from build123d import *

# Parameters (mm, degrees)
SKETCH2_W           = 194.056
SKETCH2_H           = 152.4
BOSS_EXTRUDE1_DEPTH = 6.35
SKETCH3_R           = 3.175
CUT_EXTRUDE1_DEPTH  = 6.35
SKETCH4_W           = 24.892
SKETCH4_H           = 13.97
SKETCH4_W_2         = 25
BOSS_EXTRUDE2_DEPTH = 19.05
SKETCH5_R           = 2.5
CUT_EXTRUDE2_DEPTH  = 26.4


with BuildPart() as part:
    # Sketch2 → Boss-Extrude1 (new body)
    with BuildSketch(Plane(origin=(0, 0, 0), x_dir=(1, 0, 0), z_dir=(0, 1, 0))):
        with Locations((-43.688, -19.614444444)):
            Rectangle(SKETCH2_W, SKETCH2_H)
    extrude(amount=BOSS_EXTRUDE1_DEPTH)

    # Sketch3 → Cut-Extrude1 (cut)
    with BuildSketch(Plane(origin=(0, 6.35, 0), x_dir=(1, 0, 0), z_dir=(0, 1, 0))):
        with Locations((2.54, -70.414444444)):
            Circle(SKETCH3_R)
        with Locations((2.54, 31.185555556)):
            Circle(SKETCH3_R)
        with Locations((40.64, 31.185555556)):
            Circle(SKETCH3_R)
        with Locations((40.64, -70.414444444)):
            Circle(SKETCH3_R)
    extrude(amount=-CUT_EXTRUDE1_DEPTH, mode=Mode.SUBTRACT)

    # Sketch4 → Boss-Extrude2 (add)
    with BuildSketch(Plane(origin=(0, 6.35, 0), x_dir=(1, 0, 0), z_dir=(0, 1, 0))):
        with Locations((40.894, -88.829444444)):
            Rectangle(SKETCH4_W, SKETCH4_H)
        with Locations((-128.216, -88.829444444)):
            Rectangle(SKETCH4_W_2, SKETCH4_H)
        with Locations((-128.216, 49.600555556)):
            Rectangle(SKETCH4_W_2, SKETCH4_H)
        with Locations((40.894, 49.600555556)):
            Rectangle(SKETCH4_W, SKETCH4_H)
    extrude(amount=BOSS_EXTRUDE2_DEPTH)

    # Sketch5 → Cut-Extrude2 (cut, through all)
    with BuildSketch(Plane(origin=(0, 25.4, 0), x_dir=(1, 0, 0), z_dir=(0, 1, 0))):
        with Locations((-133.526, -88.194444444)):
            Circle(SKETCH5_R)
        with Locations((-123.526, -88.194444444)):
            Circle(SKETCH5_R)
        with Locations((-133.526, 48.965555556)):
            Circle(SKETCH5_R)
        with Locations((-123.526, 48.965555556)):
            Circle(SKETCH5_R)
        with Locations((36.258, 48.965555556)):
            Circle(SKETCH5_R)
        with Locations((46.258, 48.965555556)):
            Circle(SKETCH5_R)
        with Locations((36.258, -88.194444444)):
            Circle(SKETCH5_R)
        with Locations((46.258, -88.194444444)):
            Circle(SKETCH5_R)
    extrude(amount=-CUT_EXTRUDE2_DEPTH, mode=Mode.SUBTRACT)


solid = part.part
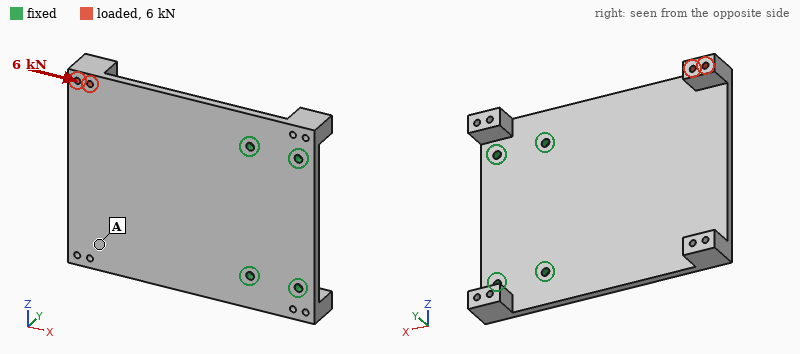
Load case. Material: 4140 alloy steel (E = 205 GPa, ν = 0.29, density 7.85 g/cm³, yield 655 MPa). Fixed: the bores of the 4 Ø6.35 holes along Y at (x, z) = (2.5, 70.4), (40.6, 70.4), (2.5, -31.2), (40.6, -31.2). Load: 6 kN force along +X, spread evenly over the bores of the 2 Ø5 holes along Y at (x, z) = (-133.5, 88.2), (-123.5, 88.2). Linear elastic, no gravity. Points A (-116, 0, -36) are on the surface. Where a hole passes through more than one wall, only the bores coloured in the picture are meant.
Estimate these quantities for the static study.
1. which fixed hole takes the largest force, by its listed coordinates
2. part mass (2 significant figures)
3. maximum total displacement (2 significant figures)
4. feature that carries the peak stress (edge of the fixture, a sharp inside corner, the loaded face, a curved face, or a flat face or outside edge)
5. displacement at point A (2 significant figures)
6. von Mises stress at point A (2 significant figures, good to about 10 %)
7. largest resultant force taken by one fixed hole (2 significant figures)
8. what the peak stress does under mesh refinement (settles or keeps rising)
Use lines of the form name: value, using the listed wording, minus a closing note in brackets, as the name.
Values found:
which fixed hole takes the largest force, by its listed coordinates: (2.5, 70.4)
part mass: 1.6 kg
maximum total displacement: 1.2 mm
feature that carries the peak stress: a sharp inside corner
displacement at point A: 0.52 mm
von Mises stress at point A: 20 MPa
largest resultant force taken by one fixed hole: 5.1 kN
what the peak stress does under mesh refinement: keeps rising
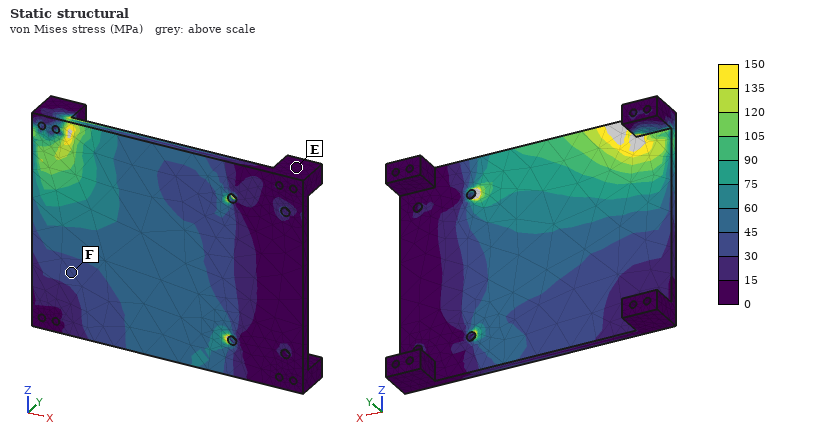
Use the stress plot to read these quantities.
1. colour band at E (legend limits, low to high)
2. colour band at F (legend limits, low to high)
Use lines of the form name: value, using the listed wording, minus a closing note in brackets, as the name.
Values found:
colour band at E: 0 to 15 MPa
colour band at F: 30 to 45 MPa
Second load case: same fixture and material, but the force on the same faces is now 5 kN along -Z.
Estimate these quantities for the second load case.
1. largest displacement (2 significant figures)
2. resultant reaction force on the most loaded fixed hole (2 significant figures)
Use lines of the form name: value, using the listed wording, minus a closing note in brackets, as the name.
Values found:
largest displacement: 0.50 mm
resultant reaction force on the most loaded fixed hole: 5.4 kN
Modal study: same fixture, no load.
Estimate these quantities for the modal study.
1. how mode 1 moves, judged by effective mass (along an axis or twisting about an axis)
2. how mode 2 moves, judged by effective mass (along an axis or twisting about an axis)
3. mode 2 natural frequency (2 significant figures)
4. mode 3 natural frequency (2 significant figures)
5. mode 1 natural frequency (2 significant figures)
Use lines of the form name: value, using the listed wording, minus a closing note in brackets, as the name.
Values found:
how mode 1 moves, judged by effective mass: along Y
how mode 2 moves, judged by effective mass: twisting about X
mode 2 natural frequency: 480 Hz
mode 3 natural frequency: 1400 Hz
mode 1 natural frequency: 220 Hz
